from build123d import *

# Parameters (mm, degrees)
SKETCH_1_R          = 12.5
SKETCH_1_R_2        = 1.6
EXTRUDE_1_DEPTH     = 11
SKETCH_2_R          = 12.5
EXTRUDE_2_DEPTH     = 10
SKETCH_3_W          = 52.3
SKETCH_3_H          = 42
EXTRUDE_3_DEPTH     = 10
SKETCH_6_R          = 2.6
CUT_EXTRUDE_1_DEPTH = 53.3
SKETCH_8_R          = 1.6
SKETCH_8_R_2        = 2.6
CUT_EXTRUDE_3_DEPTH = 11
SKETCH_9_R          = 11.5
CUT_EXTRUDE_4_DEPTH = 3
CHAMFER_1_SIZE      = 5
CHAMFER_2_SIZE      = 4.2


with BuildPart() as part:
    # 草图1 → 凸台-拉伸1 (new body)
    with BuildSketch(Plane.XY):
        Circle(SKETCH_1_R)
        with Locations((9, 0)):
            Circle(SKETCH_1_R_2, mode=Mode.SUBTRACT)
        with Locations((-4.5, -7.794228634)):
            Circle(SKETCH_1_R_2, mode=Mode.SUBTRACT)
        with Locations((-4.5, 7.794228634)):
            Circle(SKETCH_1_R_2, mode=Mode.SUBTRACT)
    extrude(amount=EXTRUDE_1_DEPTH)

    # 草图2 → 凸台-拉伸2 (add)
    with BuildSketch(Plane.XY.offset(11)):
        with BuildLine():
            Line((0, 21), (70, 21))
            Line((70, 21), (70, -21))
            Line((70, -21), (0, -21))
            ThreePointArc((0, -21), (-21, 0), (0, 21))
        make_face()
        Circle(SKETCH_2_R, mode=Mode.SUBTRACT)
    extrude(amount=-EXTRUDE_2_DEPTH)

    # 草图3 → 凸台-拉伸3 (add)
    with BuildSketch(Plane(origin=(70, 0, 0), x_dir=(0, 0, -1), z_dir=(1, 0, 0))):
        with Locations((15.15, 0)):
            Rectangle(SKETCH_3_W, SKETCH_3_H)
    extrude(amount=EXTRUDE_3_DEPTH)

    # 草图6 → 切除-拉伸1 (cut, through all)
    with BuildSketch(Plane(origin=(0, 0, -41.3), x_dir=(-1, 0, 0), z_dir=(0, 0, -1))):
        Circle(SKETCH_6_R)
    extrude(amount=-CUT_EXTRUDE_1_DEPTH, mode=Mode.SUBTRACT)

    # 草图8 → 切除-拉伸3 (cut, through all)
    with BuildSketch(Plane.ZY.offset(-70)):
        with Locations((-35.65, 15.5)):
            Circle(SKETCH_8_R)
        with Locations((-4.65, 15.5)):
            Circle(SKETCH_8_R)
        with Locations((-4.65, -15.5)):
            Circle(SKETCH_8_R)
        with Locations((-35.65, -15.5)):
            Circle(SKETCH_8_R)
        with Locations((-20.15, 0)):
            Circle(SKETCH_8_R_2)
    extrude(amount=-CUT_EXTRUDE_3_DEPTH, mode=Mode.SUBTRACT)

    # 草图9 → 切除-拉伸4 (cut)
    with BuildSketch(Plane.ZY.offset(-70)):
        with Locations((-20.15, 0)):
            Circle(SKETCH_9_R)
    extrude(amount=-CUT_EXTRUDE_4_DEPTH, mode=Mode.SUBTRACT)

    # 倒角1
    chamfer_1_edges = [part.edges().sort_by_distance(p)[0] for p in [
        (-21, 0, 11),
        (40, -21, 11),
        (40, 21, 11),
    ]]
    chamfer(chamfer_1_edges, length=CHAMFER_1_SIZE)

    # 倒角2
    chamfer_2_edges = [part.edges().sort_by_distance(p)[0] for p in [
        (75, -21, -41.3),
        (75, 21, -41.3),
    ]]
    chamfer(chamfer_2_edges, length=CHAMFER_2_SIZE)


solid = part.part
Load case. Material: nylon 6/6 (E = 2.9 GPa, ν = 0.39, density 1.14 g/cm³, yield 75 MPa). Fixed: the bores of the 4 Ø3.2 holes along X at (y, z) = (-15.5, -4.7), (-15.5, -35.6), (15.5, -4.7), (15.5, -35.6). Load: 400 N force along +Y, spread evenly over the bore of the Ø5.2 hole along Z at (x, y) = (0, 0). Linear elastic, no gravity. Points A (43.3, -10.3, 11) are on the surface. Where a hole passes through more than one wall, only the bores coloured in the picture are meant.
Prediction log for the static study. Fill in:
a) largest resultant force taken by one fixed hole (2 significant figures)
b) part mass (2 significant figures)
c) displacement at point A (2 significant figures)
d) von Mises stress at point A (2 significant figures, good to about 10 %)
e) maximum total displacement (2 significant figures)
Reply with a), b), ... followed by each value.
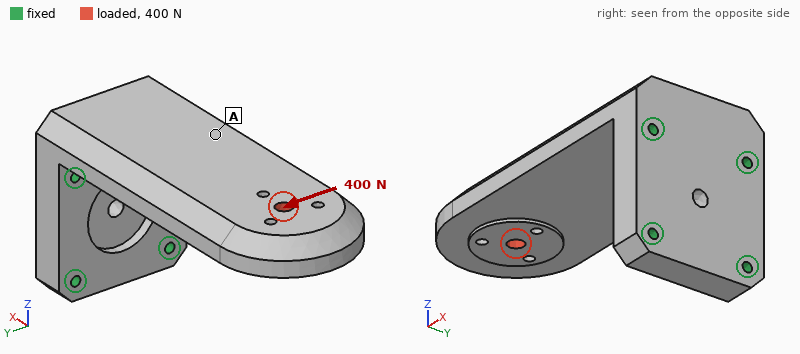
a) 940 N
b) 61 g
c) 0.31 mm
d) 3.1 MPa
e) 1.2 mm
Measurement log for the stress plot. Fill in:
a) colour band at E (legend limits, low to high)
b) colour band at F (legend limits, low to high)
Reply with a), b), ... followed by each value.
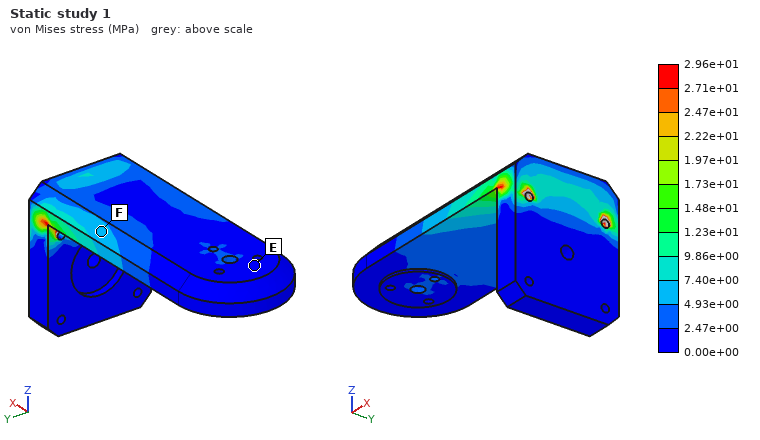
a) 0.00e+00 to 2.47e+00 MPa
b) 4.93e+00 to 7.40e+00 MPa
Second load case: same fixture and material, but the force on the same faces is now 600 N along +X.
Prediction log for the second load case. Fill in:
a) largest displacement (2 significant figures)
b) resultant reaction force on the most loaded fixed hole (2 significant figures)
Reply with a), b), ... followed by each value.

a) 0.45 mm
b) 330 N
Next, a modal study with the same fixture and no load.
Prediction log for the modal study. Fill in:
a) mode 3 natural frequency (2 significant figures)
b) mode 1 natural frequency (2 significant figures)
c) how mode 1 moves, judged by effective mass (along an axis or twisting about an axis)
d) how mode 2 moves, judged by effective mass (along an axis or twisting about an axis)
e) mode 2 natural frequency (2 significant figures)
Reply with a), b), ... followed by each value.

a) 1400 Hz
b) 260 Hz
c) along Z
d) along Y
e) 750 Hz
